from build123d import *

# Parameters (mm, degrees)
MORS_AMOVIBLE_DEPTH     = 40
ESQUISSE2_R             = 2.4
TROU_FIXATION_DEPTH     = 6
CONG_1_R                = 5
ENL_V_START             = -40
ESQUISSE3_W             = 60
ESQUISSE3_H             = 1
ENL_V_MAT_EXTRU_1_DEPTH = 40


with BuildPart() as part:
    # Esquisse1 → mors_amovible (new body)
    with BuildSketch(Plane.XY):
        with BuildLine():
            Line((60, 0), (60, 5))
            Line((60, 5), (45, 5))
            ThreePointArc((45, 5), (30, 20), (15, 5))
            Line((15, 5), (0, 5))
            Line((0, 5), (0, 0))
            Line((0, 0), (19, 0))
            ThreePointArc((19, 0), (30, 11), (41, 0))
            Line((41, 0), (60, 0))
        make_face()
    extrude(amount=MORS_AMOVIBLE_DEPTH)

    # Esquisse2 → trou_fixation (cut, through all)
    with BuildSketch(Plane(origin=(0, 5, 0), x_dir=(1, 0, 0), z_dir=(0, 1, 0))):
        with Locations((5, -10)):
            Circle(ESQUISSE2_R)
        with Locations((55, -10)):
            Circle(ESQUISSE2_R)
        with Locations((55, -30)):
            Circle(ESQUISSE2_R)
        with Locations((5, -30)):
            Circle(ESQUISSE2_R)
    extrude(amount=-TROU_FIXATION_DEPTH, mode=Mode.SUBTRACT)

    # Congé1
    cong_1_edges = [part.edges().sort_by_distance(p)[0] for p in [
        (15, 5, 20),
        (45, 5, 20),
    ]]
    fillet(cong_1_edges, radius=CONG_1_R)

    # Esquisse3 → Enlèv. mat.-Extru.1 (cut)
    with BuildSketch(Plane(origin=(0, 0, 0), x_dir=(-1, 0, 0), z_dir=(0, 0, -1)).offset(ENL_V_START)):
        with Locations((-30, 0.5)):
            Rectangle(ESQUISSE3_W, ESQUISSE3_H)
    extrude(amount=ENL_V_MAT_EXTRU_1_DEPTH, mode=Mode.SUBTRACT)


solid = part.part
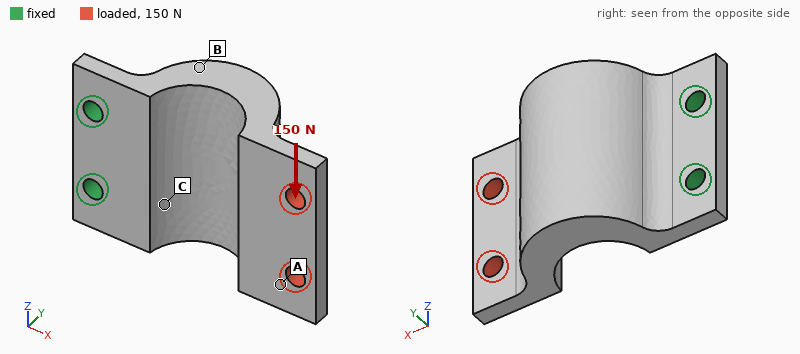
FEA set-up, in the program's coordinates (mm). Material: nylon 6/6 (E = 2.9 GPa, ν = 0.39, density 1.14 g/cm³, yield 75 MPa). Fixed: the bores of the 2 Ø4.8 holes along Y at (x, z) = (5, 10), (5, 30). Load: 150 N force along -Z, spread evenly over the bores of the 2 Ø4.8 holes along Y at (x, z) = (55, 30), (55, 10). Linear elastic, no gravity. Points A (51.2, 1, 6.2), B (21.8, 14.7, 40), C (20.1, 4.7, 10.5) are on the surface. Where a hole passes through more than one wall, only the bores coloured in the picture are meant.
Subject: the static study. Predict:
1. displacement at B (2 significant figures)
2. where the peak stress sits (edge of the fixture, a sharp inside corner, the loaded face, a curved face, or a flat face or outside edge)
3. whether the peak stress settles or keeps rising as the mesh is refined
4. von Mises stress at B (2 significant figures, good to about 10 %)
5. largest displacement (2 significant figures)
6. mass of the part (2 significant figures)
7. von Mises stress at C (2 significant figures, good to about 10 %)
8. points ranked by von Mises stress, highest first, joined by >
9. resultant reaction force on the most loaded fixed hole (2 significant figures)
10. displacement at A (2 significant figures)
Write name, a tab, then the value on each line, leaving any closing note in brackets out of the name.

displacement at B	0.27 mm
where the peak stress sits	edge of the fixture
whether the peak stress settles or keeps rising as the mesh is refined	keeps rising
von Mises stress at B	4.1 MPa
largest displacement	0.68 mm
mass of the part	19 g
von Mises stress at C	9.8 MPa
points ranked by von Mises stress, highest first, joined by >	C > B > A
resultant reaction force on the most loaded fixed hole	320 N
displacement at A	0.54 mm
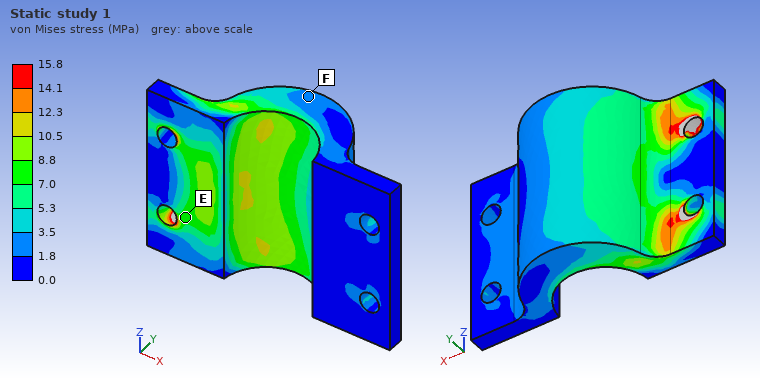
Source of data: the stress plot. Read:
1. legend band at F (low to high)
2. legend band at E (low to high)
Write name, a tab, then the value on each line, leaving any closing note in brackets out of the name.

legend band at F	1.8 to 3.5 MPa
legend band at E	7.0 to 8.8 MPa
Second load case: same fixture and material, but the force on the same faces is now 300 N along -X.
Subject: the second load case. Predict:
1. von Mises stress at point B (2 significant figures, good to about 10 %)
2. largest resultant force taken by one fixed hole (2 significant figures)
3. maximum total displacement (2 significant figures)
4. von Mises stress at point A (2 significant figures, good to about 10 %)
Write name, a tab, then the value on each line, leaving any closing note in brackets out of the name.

von Mises stress at point B	3.8 MPa
largest resultant force taken by one fixed hole	150 N
maximum total displacement	0.67 mm
von Mises stress at point A	3.0 MPa
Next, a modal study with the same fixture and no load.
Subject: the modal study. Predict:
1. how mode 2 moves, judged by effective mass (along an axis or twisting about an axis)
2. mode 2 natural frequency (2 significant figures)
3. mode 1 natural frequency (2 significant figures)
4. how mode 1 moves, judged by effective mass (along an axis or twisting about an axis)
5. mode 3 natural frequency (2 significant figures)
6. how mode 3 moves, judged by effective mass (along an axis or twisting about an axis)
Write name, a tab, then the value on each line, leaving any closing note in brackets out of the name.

how mode 2 moves, judged by effective mass	along Z
mode 2 natural frequency	1100 Hz
mode 1 natural frequency	350 Hz
how mode 1 moves, judged by effective mass	along Y
mode 3 natural frequency	1700 Hz
how mode 3 moves, judged by effective mass	along Z
